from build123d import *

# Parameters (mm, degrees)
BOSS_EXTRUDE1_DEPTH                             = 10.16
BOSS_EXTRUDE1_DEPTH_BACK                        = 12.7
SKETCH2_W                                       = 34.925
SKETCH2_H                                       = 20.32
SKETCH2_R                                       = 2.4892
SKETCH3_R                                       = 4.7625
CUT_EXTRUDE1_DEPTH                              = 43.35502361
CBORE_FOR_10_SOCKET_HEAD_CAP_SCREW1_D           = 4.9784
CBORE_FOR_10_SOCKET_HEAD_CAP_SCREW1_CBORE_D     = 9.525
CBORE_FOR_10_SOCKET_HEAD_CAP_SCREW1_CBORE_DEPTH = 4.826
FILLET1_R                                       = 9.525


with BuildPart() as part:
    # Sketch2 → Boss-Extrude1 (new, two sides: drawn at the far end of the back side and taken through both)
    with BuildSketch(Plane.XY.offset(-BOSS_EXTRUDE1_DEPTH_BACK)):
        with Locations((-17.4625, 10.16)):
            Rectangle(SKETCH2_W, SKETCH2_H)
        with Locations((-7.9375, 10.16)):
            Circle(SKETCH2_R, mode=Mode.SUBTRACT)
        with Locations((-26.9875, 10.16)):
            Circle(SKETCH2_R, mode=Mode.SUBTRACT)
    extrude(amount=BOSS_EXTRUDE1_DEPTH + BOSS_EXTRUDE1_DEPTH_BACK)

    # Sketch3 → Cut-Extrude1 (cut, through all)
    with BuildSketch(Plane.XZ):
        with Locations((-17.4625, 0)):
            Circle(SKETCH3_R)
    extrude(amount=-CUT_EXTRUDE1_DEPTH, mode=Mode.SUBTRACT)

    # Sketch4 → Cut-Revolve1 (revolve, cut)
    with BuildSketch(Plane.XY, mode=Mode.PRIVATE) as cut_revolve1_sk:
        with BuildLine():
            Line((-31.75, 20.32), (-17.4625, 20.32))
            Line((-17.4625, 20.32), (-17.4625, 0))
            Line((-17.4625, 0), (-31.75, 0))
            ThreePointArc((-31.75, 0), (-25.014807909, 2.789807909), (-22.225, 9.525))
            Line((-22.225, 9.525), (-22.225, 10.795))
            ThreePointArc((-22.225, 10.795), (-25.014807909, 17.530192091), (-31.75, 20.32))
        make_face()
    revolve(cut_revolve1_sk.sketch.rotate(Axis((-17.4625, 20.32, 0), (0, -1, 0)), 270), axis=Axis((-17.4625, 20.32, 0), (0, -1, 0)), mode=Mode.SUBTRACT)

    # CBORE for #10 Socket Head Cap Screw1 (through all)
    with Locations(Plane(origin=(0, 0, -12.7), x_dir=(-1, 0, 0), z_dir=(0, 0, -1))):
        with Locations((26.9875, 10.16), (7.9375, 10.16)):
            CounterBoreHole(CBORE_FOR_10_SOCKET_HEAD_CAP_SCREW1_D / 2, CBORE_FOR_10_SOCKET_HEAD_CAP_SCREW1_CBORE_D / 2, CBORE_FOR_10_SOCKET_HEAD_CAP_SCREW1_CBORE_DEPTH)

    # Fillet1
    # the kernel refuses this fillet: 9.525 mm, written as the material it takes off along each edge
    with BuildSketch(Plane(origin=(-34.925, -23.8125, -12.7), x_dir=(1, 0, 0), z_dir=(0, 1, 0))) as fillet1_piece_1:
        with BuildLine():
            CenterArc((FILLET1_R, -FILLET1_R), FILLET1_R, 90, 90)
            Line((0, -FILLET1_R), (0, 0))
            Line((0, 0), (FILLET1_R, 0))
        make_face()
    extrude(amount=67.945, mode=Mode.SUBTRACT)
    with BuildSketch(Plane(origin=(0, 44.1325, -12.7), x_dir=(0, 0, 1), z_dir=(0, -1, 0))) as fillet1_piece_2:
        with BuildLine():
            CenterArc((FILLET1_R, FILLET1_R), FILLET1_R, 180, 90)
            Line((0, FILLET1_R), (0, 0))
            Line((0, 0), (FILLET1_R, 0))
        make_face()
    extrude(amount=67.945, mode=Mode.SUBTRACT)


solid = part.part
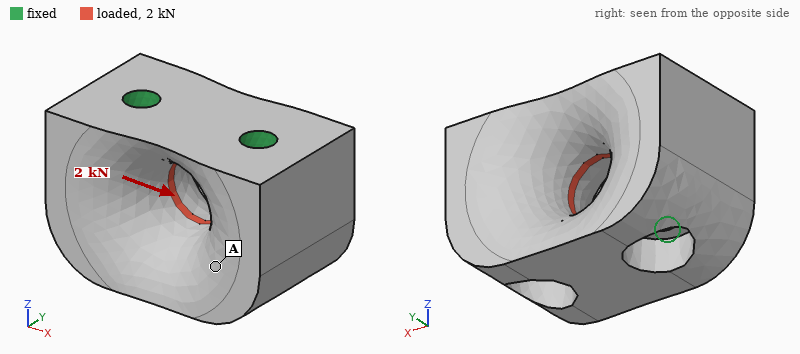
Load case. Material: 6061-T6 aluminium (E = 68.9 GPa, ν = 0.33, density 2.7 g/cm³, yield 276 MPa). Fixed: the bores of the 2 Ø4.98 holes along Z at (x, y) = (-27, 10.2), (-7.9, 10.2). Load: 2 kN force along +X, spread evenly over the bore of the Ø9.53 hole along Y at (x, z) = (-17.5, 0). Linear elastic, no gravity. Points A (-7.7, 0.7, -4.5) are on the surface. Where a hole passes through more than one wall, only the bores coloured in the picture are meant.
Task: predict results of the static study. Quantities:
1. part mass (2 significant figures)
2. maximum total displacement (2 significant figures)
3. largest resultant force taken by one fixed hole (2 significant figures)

30 g
1.8 µm
1.0 kN
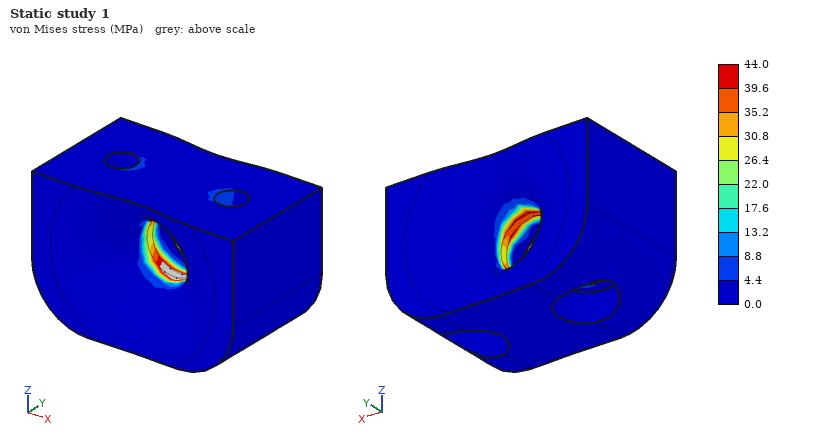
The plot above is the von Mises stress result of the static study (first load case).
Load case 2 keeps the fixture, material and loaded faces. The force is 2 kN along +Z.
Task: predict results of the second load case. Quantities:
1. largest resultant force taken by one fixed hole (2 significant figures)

1.0 kN
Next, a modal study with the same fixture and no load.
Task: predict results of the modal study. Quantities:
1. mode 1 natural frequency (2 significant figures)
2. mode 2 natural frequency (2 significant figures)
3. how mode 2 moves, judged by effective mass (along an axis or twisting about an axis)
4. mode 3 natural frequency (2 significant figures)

40 kHz
50 kHz
twisting about Z
52 kHz
